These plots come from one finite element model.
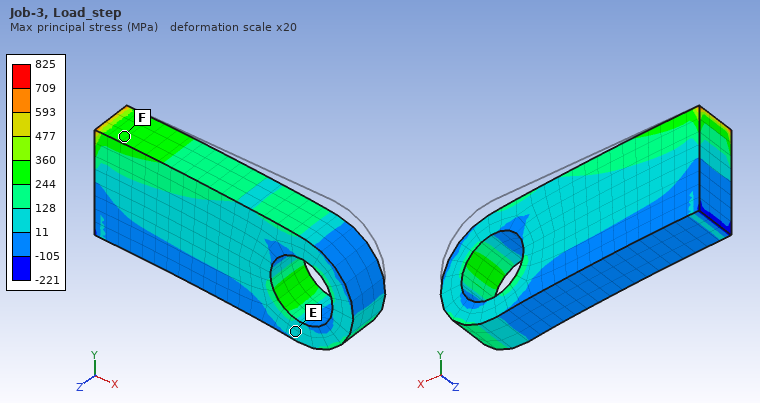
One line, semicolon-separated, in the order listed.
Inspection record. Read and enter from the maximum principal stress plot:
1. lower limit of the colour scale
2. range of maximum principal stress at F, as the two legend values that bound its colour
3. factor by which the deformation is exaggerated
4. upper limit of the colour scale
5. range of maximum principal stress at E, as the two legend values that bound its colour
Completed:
-221 MPa; 244 to 360 MPa; 20; 825 MPa; 11 to 128 MPa
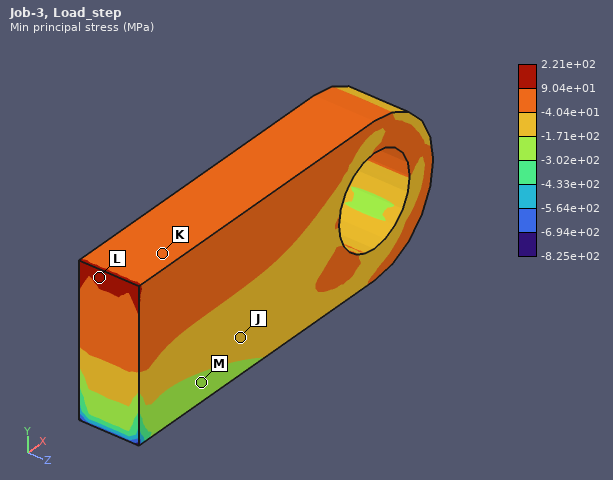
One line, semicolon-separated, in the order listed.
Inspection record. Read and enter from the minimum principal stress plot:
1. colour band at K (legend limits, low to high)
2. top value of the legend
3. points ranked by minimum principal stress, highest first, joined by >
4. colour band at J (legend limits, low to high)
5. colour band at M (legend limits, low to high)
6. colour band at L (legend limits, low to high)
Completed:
-4.04e+01 to 9.04e+01 MPa; 2.21e+02 MPa; L > K > J > M; -1.71e+02 to -4.04e+01 MPa; -3.02e+02 to -1.71e+02 MPa; 9.04e+01 to 2.21e+02 MPa
